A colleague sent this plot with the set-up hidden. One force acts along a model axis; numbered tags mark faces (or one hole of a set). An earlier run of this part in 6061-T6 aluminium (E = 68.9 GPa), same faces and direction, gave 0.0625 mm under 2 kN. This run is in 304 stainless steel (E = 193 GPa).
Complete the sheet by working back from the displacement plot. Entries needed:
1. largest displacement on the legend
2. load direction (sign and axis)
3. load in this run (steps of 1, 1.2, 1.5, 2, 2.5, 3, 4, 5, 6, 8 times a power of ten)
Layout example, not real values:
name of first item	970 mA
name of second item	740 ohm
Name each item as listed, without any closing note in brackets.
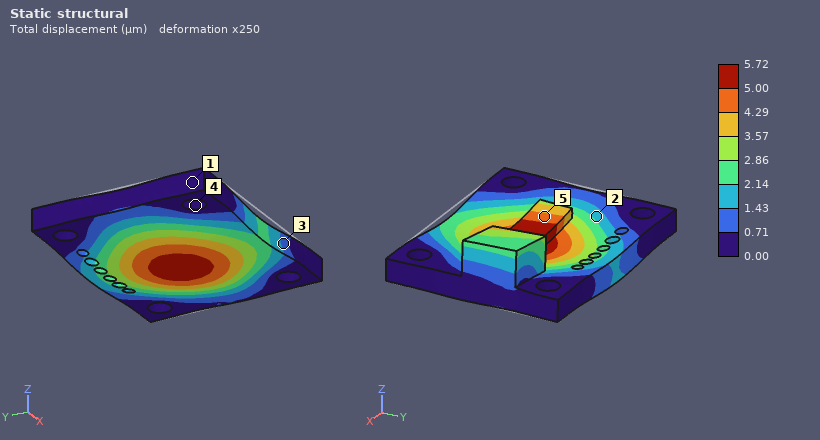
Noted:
largest displacement on the legend	5.72 µm
load direction	-Z
load in this run	500 N
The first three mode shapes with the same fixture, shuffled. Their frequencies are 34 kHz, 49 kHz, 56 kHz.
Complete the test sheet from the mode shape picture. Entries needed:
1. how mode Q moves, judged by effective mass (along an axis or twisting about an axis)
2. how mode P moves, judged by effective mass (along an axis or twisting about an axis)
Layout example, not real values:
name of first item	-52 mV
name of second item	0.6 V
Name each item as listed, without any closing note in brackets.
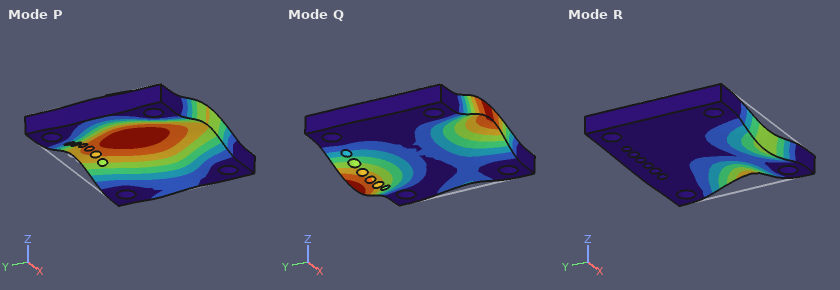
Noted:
how mode Q moves, judged by effective mass	twisting about X
how mode P moves, judged by effective mass	along Z
